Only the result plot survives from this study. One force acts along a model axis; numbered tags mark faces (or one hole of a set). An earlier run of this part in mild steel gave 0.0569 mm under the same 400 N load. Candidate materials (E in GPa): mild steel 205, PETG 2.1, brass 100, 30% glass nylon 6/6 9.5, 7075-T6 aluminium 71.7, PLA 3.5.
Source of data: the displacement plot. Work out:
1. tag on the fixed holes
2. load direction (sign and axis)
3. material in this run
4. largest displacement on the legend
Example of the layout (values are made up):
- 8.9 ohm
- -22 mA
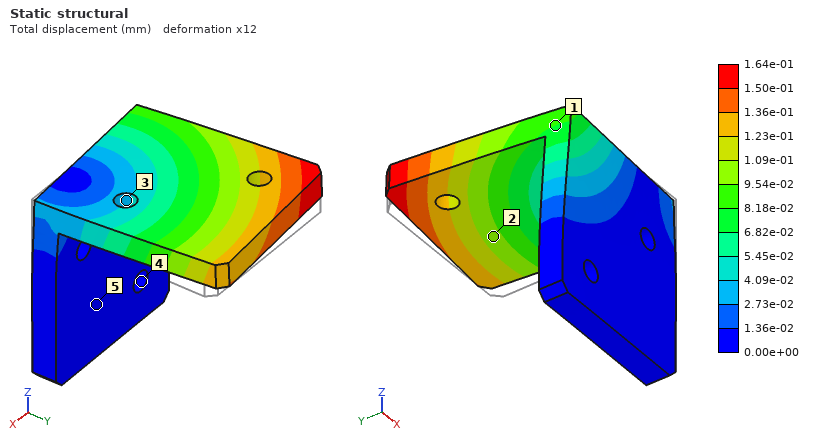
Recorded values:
- 4
- -X
- 7075-T6 aluminium
- 1.64e-01 mm
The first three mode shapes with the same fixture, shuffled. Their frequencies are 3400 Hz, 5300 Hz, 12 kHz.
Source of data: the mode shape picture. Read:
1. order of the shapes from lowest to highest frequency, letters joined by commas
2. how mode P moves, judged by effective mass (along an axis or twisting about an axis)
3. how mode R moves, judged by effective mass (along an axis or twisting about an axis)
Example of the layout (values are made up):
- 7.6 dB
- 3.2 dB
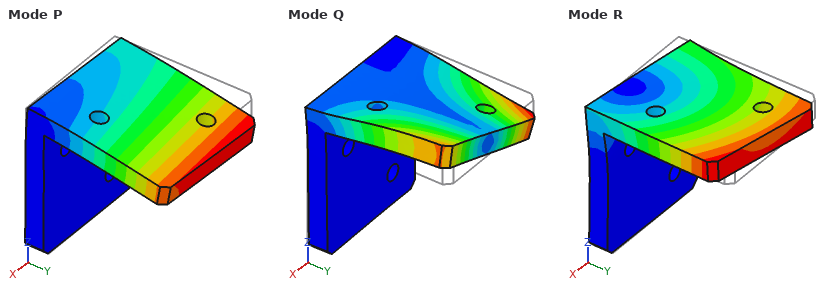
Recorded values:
- P, R, Q
- along Z
- along X
